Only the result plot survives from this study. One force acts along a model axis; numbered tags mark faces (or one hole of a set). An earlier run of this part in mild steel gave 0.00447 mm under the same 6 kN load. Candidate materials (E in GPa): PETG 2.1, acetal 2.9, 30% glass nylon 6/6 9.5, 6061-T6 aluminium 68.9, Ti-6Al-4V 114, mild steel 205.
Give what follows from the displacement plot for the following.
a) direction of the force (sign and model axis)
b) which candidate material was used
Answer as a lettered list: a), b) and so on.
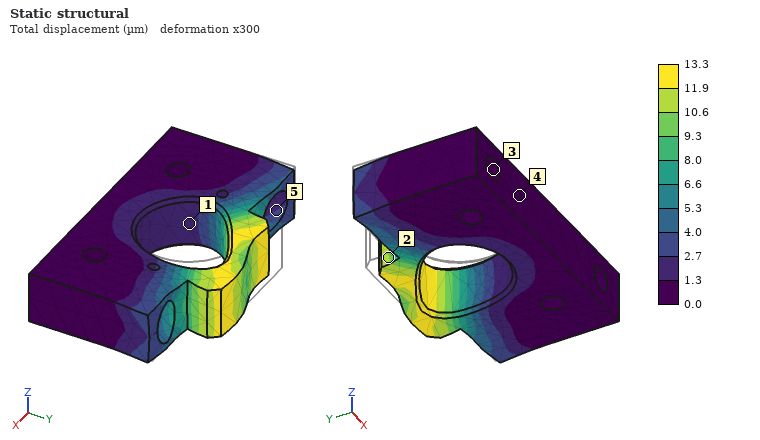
a) +X
b) 6061-T6 aluminium
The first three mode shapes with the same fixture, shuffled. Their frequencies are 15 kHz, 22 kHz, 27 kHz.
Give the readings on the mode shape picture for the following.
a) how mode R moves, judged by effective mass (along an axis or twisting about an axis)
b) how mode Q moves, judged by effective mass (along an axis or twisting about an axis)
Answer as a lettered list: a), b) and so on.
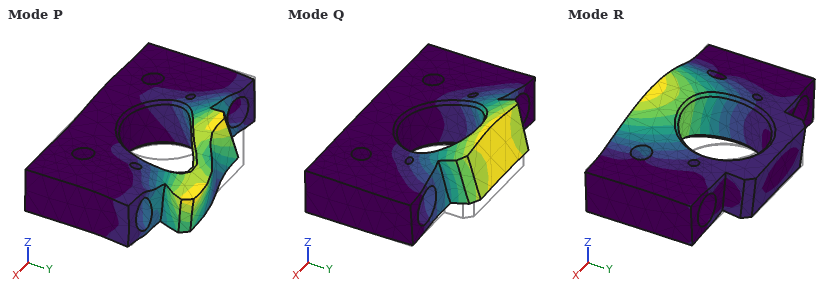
a) along Z
b) along Z
